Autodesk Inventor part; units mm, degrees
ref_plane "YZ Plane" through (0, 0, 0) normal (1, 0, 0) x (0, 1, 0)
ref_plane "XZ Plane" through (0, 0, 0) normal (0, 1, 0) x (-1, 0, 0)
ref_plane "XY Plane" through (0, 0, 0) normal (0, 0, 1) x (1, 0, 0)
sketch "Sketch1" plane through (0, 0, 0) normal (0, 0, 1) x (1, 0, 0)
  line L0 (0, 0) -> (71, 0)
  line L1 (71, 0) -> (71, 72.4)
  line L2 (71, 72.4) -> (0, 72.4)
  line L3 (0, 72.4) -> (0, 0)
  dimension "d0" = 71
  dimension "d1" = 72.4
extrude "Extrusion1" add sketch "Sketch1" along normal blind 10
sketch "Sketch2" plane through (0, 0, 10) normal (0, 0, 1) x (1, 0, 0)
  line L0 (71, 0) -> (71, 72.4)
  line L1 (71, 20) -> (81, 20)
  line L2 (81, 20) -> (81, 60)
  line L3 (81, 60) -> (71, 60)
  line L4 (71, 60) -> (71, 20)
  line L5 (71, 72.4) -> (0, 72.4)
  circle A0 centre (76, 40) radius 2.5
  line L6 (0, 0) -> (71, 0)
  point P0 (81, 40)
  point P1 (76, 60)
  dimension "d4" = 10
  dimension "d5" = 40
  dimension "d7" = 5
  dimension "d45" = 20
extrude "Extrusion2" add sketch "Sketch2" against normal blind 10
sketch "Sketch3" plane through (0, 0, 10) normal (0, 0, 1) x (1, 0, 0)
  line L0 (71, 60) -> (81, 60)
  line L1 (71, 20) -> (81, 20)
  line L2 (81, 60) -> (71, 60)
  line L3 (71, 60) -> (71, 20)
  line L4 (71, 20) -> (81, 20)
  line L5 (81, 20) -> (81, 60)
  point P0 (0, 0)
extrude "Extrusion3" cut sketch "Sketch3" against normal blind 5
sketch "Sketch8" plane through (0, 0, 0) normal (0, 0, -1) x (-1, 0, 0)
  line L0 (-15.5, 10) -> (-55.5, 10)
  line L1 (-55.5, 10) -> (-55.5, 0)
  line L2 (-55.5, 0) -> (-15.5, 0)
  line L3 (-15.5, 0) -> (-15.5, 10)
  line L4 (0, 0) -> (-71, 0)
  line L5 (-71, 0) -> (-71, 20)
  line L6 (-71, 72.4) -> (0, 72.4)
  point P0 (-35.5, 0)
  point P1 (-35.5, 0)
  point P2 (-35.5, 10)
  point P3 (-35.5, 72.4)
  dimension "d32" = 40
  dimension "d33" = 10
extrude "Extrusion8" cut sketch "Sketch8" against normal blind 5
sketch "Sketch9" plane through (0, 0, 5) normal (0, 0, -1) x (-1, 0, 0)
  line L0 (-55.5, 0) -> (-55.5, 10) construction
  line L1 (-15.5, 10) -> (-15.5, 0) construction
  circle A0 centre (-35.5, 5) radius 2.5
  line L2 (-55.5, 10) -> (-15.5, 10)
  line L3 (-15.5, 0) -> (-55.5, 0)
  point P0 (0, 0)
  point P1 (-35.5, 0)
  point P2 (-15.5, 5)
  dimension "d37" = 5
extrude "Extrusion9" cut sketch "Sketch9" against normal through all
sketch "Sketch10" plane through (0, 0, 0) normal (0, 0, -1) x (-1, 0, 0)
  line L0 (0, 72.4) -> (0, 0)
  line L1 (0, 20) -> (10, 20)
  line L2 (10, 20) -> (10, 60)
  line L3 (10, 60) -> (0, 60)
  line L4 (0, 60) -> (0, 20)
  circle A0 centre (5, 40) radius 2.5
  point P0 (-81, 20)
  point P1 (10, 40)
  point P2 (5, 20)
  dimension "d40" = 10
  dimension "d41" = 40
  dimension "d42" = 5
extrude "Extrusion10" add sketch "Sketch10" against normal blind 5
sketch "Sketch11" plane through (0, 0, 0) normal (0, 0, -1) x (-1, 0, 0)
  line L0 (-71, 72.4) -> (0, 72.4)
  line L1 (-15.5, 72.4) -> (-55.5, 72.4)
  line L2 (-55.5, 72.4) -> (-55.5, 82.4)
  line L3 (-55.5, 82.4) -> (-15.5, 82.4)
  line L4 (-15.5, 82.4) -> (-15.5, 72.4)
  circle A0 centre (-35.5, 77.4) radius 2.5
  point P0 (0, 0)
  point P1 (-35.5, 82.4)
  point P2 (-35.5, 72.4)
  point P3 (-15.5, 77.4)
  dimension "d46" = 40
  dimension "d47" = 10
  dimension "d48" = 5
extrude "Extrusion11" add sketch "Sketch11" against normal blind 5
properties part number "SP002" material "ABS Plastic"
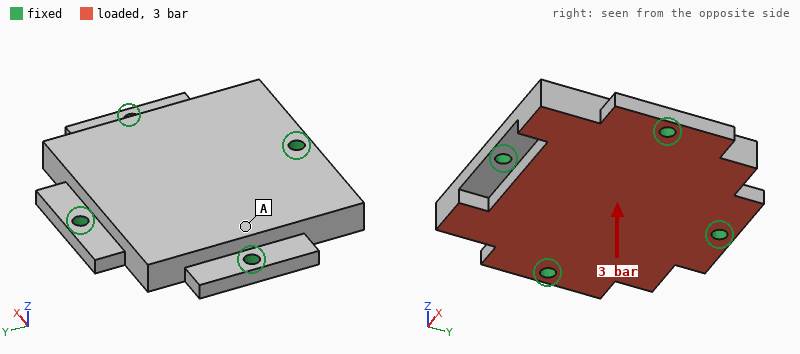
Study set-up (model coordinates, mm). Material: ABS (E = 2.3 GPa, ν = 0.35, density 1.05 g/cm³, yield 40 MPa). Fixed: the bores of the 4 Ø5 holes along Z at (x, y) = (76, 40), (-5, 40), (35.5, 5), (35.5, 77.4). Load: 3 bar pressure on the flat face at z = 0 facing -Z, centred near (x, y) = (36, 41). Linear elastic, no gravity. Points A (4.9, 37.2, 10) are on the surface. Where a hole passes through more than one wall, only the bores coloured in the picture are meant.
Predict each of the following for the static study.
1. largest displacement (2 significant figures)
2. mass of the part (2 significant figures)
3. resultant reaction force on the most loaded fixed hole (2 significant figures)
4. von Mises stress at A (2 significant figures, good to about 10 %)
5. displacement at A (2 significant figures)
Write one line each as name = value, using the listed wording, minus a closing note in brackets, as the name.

largest displacement = 0.20 mm
mass of the part = 58 g
resultant reaction force on the most loaded fixed hole = 500 N
von Mises stress at A = 5.1 MPa
displacement at A = 0.097 mm
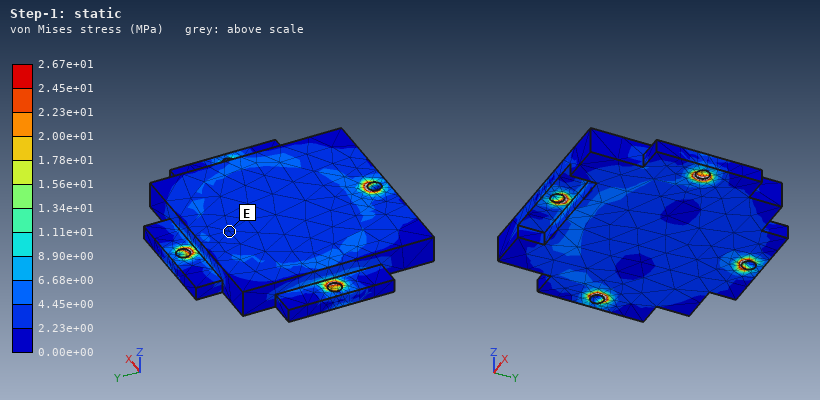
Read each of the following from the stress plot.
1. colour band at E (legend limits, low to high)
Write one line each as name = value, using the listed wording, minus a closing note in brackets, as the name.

colour band at E = 2.23e+00 to 4.45e+00 MPa
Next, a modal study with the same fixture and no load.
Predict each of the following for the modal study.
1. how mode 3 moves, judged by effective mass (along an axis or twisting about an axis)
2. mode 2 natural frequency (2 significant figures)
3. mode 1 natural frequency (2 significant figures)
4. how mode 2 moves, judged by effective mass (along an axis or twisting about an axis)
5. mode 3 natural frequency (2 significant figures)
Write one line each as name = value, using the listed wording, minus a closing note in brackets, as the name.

how mode 3 moves, judged by effective mass = along Z
mode 2 natural frequency = 2200 Hz
mode 1 natural frequency = 2000 Hz
how mode 2 moves, judged by effective mass = along Z
mode 3 natural frequency = 2400 Hz
